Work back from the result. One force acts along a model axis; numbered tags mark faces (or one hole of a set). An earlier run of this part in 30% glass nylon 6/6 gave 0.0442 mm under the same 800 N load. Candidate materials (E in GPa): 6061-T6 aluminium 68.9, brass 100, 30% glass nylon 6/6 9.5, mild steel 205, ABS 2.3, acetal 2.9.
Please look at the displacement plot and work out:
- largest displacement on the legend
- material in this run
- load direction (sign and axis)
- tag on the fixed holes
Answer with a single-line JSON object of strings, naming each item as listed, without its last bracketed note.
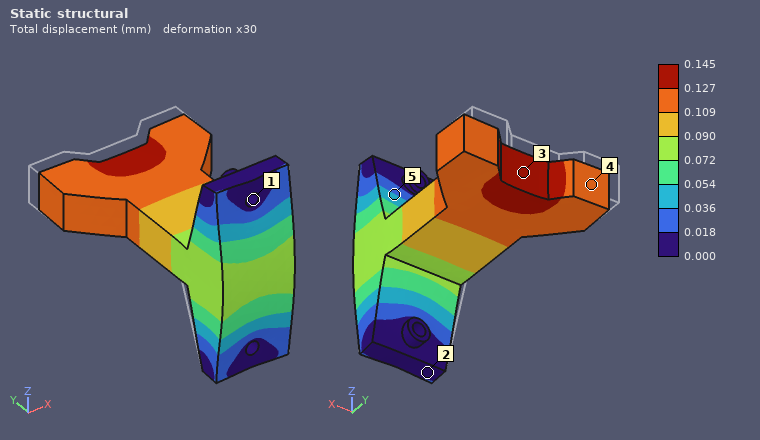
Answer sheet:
{"largest displacement on the legend": "0.145 mm", "material in this run": "acetal", "load direction": "-Y", "tag on the fixed holes": "1"}
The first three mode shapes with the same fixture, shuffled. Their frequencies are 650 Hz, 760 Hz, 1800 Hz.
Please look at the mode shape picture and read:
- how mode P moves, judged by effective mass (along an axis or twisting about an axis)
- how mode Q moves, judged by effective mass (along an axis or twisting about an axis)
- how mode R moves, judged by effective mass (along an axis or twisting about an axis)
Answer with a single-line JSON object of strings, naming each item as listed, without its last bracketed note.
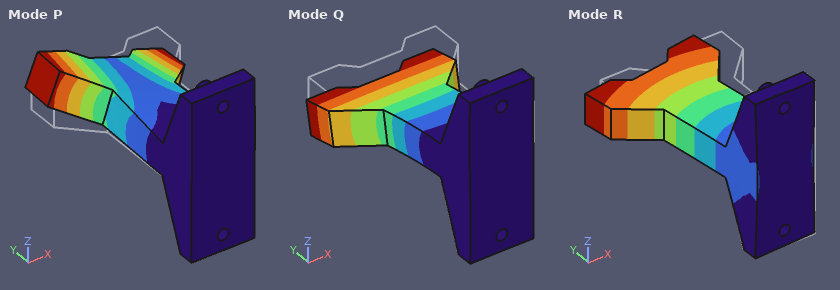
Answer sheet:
{"how mode P moves, judged by effective mass": "twisting about Y", "how mode Q moves, judged by effective mass": "along Z", "how mode R moves, judged by effective mass": "along X"}
